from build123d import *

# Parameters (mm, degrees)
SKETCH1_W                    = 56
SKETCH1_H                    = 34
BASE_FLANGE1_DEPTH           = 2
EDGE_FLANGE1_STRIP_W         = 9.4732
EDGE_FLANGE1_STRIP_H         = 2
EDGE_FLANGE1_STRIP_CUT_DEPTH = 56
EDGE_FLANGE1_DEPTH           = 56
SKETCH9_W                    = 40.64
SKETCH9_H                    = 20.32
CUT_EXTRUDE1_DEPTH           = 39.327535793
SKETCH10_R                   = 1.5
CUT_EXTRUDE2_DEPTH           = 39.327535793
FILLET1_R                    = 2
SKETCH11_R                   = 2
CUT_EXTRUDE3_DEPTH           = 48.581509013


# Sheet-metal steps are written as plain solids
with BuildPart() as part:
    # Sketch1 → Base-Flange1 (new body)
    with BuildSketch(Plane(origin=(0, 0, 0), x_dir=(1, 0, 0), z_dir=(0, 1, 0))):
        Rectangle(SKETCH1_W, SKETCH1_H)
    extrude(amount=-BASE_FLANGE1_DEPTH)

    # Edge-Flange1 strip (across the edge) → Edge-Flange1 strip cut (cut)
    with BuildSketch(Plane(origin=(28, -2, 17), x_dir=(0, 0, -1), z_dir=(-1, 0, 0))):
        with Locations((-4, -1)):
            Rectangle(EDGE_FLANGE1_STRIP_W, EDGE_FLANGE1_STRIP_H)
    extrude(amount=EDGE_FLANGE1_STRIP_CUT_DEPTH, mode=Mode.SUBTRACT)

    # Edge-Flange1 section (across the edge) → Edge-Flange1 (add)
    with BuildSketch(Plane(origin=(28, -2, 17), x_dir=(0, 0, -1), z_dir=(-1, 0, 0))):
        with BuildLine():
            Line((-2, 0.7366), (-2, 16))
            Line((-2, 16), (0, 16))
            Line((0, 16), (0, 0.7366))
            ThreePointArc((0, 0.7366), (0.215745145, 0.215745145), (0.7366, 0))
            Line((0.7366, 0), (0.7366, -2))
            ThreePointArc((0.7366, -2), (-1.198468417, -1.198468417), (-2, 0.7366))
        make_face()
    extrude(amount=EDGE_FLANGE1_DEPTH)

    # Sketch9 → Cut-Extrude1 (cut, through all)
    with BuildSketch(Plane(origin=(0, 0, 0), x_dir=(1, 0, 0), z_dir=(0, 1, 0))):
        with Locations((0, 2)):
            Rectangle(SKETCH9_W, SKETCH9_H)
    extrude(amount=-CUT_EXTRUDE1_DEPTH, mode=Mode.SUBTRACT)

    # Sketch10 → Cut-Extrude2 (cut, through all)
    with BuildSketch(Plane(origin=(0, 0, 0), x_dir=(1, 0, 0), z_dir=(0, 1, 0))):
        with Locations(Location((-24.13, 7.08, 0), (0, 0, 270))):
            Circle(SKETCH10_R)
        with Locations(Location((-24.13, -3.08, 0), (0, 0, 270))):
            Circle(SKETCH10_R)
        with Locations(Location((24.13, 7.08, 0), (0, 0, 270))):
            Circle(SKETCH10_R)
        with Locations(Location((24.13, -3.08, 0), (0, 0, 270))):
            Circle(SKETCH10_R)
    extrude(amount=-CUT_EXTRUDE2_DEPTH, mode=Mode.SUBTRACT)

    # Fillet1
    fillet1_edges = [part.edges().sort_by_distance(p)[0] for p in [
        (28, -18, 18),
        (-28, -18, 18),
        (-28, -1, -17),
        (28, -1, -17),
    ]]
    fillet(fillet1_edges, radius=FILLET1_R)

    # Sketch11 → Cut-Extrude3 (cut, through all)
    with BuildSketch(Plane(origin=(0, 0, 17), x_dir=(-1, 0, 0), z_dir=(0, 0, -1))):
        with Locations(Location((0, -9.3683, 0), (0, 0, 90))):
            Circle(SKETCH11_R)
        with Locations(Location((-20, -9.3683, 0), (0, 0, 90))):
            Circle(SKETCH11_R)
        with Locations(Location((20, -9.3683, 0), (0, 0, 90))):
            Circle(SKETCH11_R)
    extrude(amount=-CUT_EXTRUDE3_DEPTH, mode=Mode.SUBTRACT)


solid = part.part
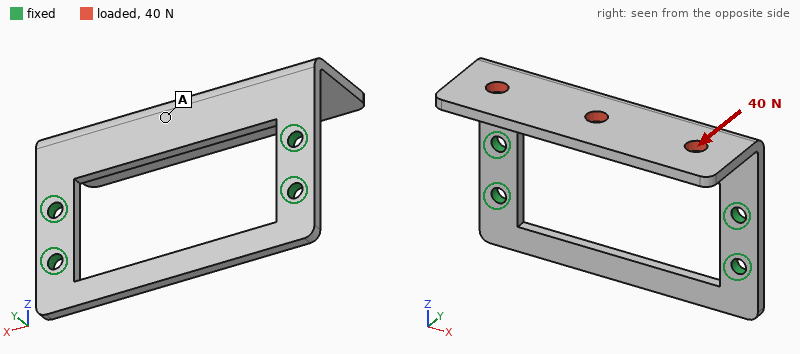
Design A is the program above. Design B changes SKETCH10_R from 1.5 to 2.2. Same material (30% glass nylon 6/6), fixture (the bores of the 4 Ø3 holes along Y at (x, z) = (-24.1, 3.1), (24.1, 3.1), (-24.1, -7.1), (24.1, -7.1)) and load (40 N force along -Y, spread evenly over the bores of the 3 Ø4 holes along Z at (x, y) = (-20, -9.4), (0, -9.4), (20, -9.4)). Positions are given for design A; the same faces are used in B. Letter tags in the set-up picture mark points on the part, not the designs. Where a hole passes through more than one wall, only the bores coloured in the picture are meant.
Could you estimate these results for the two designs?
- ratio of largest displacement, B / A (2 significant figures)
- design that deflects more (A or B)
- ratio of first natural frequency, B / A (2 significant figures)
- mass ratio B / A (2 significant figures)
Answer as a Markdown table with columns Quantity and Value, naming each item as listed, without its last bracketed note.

| Quantity | Value |
|---|---|
| ratio of largest displacement, B / A | 0.85 |
| design that deflects more | A |
| ratio of first natural frequency, B / A | 1.1 |
| mass ratio B / A | 0.98 |
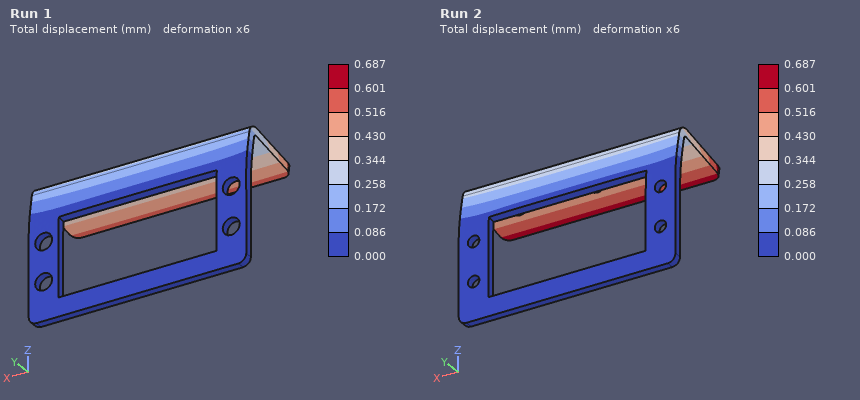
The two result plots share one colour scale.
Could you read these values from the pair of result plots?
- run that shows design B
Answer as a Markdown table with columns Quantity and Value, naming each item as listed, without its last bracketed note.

| Quantity | Value |
|---|---|
| run that shows design B | Run 1 |
